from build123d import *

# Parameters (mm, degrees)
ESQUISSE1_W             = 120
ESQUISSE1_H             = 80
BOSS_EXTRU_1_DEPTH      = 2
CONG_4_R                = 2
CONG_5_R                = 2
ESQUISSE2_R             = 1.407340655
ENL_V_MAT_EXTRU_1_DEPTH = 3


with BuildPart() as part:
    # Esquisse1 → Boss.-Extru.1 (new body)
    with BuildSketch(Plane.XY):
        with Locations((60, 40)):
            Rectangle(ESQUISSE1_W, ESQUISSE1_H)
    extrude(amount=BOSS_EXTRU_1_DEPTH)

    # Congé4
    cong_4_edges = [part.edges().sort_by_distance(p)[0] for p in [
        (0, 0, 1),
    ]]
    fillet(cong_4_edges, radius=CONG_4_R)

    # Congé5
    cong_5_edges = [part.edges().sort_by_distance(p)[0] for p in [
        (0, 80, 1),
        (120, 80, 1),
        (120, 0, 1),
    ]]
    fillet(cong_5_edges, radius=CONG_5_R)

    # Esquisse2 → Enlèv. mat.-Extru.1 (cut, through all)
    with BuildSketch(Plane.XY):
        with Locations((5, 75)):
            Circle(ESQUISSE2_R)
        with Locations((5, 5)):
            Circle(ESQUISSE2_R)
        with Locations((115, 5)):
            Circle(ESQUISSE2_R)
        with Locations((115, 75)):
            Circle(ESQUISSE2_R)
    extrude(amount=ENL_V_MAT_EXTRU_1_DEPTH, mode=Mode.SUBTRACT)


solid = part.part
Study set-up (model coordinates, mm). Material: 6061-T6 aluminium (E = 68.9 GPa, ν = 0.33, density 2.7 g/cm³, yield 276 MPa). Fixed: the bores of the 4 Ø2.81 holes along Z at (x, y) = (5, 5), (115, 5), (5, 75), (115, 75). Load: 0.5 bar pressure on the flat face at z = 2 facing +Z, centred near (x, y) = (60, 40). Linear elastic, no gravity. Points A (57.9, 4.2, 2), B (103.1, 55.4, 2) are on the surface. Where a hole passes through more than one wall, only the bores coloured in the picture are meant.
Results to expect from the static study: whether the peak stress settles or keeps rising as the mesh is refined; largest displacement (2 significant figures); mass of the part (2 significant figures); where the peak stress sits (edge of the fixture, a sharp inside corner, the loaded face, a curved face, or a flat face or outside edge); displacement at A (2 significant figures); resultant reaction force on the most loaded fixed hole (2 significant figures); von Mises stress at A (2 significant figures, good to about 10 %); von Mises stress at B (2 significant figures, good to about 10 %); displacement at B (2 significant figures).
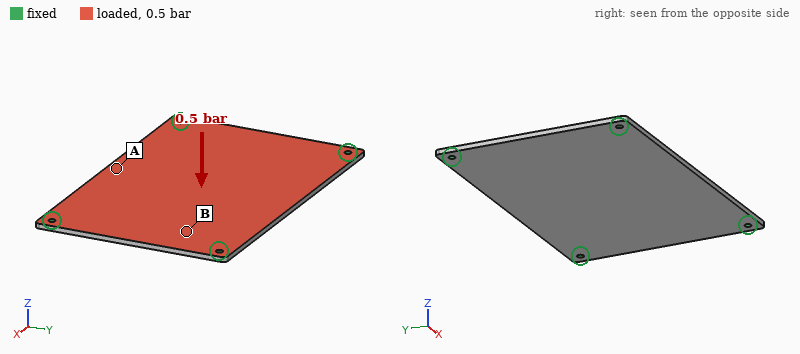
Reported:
keeps rising
0.68 mm
52 g
edge of the fixture
0.63 mm
120 N
52 MPa
20 MPa
0.23 mm
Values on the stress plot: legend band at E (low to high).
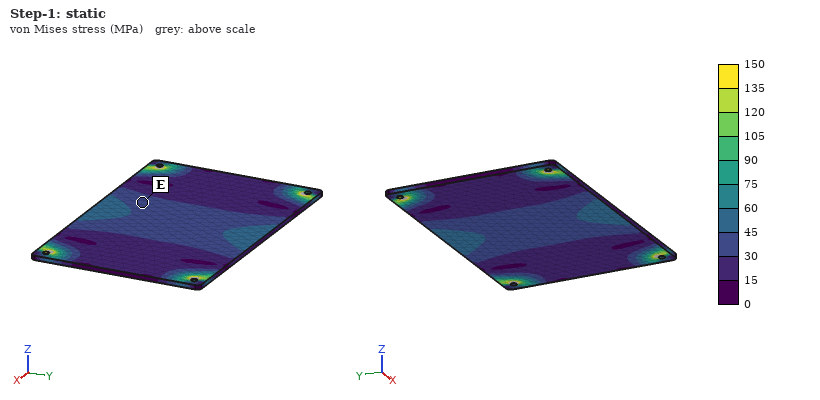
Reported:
30 to 45 MPa
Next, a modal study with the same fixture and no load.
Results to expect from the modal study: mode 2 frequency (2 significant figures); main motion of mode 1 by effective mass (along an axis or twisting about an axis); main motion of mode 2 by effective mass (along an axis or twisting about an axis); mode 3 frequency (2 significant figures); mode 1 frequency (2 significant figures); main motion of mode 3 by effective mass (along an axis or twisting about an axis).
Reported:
1100 Hz
along Z
twisting about X
1700 Hz
680 Hz
twisting about Y
